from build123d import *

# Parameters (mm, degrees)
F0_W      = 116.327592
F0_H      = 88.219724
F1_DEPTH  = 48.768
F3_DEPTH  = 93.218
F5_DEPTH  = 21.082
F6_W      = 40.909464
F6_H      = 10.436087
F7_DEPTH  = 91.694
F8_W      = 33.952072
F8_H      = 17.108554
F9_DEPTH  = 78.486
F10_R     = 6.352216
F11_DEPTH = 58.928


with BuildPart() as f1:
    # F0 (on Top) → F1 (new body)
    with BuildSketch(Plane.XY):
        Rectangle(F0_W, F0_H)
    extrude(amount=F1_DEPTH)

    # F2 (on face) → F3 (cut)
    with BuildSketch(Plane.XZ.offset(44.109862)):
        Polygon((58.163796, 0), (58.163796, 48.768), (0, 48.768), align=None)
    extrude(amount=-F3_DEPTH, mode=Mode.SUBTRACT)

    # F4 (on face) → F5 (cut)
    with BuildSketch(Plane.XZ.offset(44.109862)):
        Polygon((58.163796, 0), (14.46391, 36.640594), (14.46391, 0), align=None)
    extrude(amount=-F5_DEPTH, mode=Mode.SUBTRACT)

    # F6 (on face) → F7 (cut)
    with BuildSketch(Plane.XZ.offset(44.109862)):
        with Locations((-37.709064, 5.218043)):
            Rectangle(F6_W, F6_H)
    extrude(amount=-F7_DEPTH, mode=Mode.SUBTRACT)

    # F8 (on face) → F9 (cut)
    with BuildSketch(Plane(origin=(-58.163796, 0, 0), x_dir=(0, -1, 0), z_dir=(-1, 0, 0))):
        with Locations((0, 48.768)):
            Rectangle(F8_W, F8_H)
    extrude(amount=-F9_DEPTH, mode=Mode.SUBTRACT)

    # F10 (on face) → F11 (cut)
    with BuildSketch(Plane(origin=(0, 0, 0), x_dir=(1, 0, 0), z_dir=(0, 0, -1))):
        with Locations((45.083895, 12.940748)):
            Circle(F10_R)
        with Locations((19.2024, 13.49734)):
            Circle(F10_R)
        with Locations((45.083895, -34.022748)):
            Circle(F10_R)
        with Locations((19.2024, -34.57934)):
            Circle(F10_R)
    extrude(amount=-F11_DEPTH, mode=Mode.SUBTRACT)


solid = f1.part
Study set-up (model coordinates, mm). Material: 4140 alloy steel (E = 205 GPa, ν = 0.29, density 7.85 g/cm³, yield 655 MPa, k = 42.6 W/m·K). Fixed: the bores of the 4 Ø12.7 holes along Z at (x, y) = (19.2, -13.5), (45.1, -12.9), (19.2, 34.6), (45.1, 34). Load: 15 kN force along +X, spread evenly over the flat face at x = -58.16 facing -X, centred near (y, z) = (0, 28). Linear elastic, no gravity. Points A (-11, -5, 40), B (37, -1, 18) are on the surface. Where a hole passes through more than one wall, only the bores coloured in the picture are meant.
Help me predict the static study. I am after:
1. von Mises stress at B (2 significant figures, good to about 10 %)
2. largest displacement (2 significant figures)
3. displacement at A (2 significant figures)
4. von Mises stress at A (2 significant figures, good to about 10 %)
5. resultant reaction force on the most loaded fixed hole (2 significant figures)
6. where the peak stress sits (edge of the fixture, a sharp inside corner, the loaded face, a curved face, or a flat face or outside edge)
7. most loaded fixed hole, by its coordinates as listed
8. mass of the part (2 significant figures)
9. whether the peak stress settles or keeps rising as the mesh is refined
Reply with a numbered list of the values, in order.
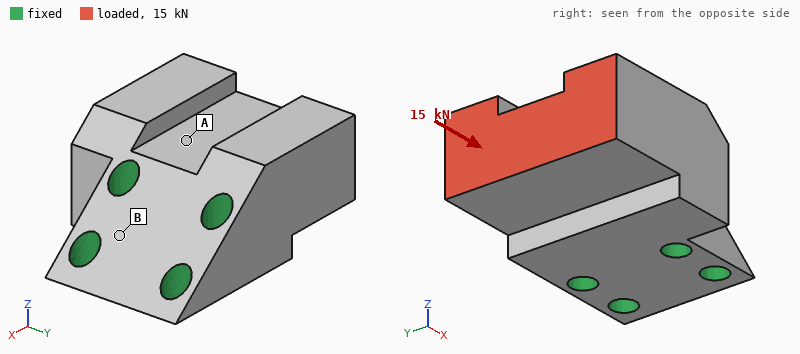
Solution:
1. 3.1 MPa
2. 6.2 µm
3. 2.3 µm
4. 8.5 MPa
5. 10 kN
6. edge of the fixture
7. (19.2, -13.5)
8. 2.3 kg
9. keeps rising
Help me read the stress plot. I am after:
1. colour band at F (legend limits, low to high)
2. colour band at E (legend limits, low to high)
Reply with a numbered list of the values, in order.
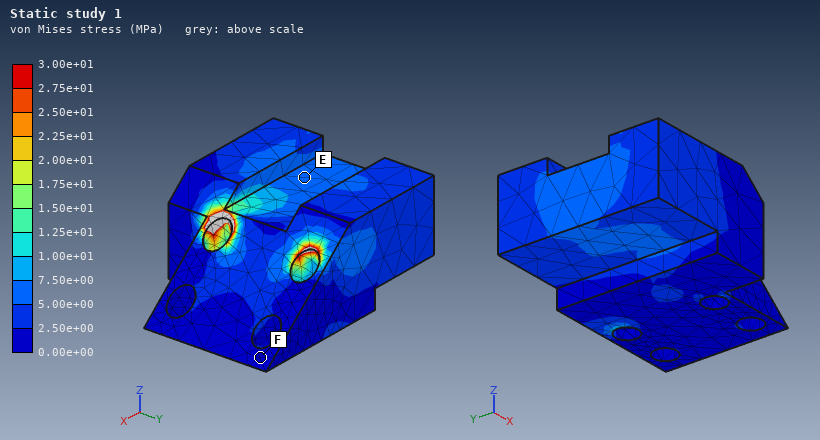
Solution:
1. 0.00e+00 to 2.50e+00 MPa
2. 5.00e+00 to 7.50e+00 MPa
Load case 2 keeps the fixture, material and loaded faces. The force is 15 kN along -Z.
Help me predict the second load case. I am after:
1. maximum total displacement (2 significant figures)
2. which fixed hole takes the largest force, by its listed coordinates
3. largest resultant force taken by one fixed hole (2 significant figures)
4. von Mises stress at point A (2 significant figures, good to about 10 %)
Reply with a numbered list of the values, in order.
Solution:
1. 45 µm
2. (19.2, -13.5)
3. 9.8 kN
4. 32 MPa
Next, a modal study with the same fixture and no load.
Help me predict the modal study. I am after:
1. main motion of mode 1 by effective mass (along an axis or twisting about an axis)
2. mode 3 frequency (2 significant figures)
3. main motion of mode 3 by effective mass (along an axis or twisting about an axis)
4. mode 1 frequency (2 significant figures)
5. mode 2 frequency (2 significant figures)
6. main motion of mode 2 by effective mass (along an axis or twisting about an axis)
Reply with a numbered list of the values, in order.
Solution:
1. along Z
2. 6900 Hz
3. twisting about X
4. 4200 Hz
5. 5900 Hz
6. along Y
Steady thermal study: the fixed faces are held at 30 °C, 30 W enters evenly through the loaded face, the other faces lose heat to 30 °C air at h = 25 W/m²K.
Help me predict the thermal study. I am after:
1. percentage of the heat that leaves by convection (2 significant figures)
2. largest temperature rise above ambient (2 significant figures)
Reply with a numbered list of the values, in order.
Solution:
1. 15 %
2. 16 K
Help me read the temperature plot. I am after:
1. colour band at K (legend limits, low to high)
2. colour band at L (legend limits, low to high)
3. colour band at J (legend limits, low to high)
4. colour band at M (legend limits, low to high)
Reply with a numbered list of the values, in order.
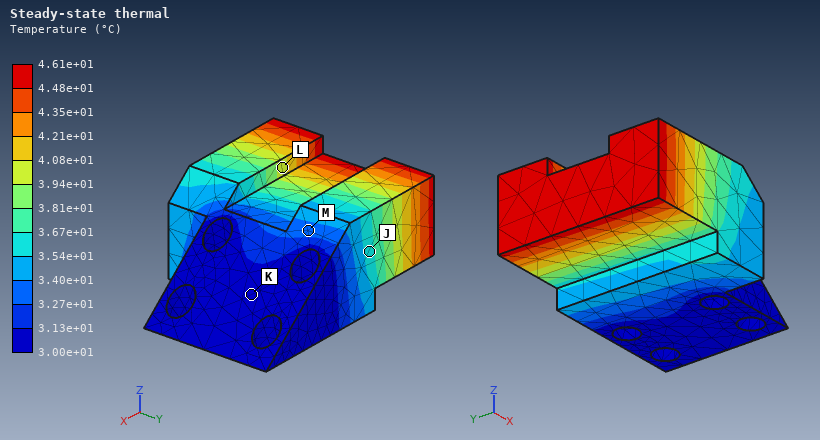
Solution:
1. 3.00e+01 to 3.13e+01 °C
2. 3.94e+01 to 4.08e+01 °C
3. 3.54e+01 to 3.67e+01 °C
4. 3.27e+01 to 3.40e+01 °C
